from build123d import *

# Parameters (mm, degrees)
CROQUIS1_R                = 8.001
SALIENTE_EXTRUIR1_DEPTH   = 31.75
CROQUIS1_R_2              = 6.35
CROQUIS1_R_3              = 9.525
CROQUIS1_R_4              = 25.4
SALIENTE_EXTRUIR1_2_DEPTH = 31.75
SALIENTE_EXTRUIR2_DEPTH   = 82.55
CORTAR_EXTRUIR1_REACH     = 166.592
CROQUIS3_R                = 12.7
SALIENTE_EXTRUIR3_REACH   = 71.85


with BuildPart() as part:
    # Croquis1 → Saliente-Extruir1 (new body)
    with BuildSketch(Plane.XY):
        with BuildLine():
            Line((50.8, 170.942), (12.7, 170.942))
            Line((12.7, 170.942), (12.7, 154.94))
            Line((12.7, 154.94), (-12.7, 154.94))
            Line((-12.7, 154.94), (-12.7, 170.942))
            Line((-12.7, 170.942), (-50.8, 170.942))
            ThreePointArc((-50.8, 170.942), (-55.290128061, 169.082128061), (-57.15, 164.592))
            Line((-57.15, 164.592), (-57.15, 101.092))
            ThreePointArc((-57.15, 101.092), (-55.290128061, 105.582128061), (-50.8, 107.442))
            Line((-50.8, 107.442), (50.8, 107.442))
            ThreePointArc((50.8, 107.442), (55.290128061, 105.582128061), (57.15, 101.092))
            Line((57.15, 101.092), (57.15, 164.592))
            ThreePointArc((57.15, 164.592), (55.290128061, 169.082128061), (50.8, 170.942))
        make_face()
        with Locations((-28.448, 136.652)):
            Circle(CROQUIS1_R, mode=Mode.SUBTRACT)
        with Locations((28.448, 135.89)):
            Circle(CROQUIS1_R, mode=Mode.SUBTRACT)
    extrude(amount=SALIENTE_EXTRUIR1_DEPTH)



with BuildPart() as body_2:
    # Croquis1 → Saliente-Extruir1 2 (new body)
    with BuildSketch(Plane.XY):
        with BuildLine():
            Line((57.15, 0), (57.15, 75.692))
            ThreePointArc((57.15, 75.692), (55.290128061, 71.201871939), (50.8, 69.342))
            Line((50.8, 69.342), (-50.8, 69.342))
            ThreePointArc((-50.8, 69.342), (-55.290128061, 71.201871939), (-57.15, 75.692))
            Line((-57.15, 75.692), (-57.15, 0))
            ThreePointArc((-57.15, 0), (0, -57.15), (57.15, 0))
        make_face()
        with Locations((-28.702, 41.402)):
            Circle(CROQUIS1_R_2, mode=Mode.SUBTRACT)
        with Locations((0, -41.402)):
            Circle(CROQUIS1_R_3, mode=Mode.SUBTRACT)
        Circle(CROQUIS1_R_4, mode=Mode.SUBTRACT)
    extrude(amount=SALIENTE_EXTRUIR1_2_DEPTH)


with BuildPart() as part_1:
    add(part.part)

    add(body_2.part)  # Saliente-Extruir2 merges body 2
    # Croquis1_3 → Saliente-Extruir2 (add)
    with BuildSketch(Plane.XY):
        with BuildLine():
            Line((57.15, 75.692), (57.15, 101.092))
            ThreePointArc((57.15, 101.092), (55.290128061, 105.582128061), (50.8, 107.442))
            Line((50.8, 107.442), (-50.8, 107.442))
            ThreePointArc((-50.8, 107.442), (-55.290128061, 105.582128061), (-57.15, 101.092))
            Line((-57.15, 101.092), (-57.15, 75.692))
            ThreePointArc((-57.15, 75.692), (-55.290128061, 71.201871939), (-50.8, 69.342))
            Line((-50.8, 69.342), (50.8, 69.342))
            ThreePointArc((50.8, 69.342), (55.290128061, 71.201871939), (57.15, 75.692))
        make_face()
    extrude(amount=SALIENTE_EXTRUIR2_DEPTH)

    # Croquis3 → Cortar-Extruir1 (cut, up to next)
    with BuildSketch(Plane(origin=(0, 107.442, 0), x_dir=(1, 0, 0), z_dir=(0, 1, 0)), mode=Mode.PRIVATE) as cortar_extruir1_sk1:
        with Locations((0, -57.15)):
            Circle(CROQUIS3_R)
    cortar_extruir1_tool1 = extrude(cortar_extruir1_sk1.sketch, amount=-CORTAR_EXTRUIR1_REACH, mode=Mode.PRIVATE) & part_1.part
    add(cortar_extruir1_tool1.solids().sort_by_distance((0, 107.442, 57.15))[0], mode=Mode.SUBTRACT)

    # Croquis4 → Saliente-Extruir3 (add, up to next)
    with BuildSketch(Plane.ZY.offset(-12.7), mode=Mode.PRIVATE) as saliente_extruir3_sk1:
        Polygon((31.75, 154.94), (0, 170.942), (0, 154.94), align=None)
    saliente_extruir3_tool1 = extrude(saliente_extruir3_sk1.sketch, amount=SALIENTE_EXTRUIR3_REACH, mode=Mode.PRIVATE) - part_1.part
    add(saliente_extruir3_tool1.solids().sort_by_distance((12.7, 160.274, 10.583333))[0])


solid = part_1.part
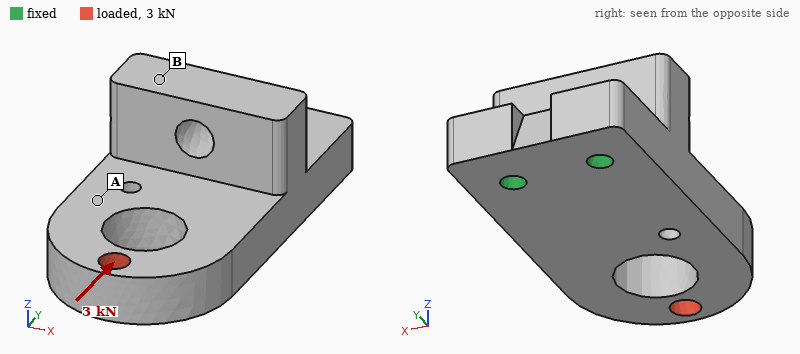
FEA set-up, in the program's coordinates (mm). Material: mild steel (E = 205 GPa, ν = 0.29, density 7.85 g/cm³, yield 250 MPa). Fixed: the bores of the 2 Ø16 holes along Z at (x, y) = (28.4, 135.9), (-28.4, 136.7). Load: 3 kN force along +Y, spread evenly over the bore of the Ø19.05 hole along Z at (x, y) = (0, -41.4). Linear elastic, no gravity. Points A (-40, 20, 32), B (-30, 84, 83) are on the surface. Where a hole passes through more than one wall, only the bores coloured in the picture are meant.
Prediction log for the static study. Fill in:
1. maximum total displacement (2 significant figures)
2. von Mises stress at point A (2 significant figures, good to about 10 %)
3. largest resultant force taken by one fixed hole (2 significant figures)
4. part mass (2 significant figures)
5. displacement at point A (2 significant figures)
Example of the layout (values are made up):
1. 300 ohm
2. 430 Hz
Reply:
1. 2.3 µm
2. 2.2 MPa
3. 1.5 kN
4. 7.0 kg
5. 0.73 µm
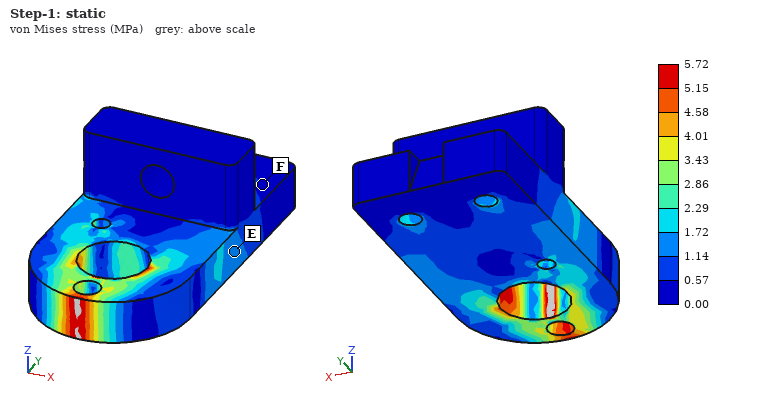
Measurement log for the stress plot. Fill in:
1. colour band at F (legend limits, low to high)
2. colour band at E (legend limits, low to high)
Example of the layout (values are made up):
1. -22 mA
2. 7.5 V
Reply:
1. 0.00 to 0.57 MPa
2. 1.14 to 1.72 MPa
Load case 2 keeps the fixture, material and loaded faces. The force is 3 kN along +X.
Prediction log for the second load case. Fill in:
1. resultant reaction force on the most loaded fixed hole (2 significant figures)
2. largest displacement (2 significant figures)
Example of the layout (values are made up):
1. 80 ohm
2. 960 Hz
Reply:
1. 8.0 kN
2. 14 µm
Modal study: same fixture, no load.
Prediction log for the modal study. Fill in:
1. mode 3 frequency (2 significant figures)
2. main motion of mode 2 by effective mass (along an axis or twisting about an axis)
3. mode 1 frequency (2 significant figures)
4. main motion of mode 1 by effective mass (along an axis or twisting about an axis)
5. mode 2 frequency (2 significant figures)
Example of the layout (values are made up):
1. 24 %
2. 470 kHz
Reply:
1. 2600 Hz
2. along X
3. 880 Hz
4. along Z
5. 2200 Hz
